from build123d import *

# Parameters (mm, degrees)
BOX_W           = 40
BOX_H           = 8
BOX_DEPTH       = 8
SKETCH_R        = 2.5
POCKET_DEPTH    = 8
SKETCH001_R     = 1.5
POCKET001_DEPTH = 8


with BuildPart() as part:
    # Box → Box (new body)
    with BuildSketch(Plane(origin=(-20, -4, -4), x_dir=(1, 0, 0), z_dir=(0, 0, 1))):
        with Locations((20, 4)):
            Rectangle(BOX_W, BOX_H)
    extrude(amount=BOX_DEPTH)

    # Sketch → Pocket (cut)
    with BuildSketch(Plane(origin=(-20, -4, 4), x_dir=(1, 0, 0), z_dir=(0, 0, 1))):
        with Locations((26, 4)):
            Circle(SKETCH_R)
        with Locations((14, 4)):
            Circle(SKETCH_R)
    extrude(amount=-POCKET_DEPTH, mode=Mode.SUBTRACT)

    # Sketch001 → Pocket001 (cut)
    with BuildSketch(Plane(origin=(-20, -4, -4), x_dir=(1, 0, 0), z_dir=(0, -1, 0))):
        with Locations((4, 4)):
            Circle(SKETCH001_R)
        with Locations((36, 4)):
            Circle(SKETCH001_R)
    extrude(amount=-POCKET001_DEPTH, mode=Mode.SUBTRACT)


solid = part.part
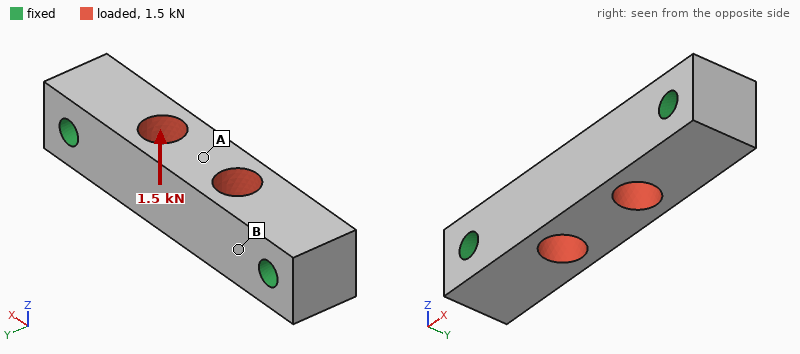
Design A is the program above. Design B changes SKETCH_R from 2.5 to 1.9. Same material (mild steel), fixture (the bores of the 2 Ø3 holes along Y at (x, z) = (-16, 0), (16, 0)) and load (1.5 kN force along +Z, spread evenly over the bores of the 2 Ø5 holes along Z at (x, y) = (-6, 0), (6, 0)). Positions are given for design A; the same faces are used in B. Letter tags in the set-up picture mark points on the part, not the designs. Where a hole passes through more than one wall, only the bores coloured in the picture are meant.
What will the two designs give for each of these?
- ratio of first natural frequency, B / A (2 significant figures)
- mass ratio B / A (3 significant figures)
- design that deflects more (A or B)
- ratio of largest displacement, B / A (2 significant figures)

1.1
1.06
A
0.90
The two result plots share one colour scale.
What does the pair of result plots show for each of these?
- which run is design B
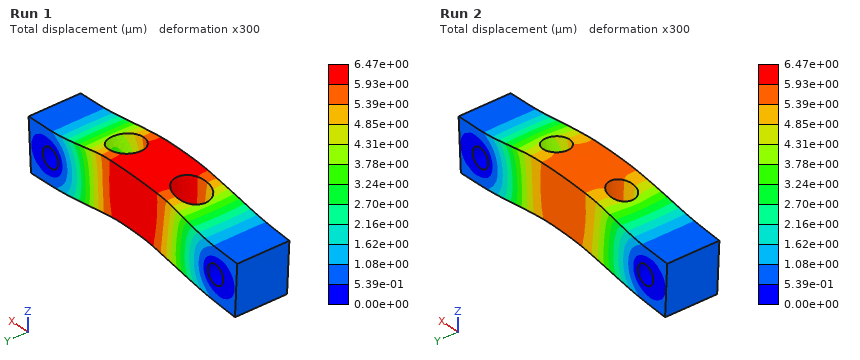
Run 2
